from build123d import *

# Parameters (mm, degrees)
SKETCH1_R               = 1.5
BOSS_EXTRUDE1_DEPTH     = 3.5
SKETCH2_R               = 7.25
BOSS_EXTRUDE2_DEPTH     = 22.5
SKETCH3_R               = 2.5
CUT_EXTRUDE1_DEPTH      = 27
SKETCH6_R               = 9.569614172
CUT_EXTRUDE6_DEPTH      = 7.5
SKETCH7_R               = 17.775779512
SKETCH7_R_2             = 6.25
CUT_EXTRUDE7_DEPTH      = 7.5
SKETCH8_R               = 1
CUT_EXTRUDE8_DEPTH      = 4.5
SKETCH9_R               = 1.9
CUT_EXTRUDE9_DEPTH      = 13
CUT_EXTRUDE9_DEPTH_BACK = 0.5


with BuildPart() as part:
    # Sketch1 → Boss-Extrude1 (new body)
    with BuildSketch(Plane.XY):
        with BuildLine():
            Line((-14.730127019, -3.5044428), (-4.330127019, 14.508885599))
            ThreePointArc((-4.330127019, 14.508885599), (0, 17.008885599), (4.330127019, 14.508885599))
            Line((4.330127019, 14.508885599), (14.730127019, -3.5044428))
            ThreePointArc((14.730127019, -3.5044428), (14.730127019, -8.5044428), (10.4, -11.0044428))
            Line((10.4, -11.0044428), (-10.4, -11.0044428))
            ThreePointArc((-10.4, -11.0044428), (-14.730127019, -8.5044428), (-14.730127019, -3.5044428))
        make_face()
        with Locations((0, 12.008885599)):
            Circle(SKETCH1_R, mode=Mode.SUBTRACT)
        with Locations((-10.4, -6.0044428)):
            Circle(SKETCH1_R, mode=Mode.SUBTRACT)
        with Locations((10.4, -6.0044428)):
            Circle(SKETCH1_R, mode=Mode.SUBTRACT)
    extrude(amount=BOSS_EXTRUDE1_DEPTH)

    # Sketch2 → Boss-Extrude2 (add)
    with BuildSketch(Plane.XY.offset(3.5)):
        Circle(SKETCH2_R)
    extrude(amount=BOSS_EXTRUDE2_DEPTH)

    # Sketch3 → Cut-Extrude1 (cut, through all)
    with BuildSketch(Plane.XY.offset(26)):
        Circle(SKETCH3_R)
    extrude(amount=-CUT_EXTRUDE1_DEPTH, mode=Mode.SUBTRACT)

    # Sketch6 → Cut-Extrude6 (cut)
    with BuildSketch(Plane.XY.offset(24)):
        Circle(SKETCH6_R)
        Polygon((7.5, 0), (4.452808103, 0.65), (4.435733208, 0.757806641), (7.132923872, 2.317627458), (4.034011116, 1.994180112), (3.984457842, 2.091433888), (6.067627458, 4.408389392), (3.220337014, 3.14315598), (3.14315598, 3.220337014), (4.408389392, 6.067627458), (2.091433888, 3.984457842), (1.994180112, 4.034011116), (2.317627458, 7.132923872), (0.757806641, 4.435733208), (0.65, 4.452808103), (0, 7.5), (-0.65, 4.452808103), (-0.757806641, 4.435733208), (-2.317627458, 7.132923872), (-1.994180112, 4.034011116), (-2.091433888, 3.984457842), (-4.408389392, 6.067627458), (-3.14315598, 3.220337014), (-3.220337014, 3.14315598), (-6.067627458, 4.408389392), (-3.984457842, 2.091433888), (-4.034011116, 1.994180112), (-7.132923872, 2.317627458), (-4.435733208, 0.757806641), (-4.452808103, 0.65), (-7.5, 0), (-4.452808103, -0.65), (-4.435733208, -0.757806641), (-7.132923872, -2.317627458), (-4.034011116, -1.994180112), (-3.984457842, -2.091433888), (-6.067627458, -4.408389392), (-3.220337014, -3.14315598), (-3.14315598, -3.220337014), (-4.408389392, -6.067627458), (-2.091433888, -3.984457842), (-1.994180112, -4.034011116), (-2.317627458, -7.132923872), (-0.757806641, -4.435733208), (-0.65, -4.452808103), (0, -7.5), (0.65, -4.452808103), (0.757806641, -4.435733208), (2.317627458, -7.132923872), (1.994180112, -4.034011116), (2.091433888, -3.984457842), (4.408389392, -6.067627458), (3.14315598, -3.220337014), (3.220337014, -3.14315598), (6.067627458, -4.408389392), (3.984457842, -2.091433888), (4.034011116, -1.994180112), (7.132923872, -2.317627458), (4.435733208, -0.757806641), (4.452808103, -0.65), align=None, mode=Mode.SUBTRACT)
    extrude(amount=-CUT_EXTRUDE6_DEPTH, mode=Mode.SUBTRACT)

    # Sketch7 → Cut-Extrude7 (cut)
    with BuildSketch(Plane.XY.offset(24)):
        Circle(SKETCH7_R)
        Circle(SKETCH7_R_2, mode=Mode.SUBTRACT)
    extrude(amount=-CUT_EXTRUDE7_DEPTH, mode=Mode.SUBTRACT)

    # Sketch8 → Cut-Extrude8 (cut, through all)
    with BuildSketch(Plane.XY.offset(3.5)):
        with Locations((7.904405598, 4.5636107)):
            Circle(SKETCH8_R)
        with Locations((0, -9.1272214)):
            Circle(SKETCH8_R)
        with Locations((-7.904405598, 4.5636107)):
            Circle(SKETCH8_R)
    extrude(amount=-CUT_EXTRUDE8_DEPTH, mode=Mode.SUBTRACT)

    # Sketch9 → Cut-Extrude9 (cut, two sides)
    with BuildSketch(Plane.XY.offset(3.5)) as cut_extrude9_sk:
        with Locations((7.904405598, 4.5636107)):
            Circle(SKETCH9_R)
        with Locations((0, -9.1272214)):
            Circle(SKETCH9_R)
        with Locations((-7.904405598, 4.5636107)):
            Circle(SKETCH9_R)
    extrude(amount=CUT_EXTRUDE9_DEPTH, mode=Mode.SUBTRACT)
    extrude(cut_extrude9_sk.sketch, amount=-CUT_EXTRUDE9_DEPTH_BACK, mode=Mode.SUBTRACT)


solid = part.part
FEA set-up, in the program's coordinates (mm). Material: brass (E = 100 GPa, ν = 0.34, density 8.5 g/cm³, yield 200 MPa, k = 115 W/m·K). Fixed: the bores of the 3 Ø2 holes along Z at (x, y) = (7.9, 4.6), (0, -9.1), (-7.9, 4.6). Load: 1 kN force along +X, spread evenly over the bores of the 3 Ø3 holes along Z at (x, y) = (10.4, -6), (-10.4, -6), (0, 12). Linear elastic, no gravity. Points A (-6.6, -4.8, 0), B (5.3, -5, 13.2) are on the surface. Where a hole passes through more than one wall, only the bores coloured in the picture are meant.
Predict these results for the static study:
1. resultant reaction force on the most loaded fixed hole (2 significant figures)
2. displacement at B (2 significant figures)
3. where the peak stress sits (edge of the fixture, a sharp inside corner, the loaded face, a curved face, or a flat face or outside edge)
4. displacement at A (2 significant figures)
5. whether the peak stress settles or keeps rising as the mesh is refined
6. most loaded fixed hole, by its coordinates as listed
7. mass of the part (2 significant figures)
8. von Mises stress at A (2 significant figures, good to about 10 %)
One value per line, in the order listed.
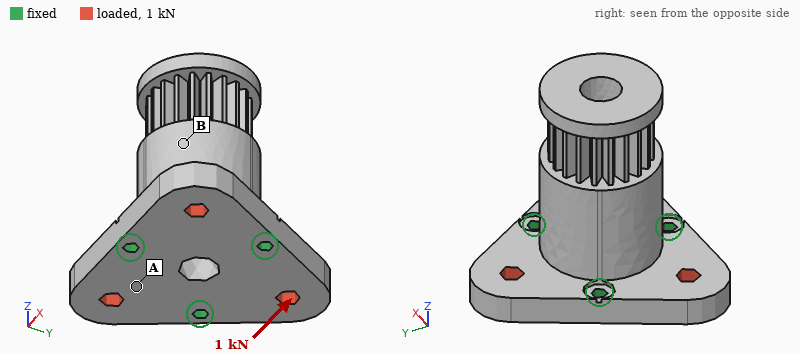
480 N
0.47 µm
edge of the fixture
1.0 µm
keeps rising
(0, -9.1)
39 g
9.0 MPa
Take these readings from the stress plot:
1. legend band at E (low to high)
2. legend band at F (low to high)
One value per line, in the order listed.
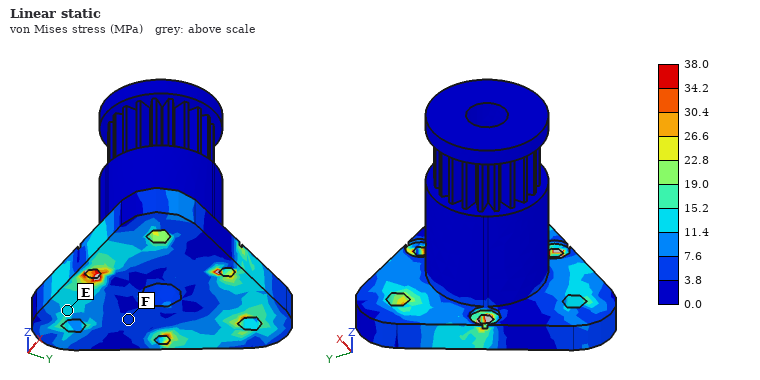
11.4 to 15.2 MPa
3.8 to 7.6 MPa
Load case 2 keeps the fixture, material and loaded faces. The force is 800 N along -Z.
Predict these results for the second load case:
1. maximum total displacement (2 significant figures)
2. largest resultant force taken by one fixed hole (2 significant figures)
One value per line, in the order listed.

15 µm
280 N
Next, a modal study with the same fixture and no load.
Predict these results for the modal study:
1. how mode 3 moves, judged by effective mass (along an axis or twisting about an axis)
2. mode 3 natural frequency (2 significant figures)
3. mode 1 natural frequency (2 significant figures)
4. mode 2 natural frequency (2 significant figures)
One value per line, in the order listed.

along Z
16 kHz
7800 Hz
7800 Hz
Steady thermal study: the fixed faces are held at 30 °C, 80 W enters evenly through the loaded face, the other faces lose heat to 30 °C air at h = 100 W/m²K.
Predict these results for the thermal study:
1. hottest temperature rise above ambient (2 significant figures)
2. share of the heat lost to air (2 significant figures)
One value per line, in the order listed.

58 K
9.2 %
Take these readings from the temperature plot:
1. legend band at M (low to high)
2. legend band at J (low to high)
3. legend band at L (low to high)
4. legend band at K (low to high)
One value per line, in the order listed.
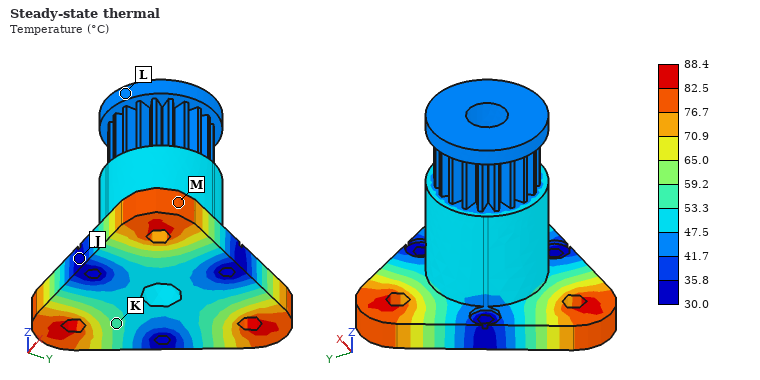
76.7 to 82.5 °C
30.0 to 35.8 °C
41.7 to 47.5 °C
53.3 to 59.2 °C
